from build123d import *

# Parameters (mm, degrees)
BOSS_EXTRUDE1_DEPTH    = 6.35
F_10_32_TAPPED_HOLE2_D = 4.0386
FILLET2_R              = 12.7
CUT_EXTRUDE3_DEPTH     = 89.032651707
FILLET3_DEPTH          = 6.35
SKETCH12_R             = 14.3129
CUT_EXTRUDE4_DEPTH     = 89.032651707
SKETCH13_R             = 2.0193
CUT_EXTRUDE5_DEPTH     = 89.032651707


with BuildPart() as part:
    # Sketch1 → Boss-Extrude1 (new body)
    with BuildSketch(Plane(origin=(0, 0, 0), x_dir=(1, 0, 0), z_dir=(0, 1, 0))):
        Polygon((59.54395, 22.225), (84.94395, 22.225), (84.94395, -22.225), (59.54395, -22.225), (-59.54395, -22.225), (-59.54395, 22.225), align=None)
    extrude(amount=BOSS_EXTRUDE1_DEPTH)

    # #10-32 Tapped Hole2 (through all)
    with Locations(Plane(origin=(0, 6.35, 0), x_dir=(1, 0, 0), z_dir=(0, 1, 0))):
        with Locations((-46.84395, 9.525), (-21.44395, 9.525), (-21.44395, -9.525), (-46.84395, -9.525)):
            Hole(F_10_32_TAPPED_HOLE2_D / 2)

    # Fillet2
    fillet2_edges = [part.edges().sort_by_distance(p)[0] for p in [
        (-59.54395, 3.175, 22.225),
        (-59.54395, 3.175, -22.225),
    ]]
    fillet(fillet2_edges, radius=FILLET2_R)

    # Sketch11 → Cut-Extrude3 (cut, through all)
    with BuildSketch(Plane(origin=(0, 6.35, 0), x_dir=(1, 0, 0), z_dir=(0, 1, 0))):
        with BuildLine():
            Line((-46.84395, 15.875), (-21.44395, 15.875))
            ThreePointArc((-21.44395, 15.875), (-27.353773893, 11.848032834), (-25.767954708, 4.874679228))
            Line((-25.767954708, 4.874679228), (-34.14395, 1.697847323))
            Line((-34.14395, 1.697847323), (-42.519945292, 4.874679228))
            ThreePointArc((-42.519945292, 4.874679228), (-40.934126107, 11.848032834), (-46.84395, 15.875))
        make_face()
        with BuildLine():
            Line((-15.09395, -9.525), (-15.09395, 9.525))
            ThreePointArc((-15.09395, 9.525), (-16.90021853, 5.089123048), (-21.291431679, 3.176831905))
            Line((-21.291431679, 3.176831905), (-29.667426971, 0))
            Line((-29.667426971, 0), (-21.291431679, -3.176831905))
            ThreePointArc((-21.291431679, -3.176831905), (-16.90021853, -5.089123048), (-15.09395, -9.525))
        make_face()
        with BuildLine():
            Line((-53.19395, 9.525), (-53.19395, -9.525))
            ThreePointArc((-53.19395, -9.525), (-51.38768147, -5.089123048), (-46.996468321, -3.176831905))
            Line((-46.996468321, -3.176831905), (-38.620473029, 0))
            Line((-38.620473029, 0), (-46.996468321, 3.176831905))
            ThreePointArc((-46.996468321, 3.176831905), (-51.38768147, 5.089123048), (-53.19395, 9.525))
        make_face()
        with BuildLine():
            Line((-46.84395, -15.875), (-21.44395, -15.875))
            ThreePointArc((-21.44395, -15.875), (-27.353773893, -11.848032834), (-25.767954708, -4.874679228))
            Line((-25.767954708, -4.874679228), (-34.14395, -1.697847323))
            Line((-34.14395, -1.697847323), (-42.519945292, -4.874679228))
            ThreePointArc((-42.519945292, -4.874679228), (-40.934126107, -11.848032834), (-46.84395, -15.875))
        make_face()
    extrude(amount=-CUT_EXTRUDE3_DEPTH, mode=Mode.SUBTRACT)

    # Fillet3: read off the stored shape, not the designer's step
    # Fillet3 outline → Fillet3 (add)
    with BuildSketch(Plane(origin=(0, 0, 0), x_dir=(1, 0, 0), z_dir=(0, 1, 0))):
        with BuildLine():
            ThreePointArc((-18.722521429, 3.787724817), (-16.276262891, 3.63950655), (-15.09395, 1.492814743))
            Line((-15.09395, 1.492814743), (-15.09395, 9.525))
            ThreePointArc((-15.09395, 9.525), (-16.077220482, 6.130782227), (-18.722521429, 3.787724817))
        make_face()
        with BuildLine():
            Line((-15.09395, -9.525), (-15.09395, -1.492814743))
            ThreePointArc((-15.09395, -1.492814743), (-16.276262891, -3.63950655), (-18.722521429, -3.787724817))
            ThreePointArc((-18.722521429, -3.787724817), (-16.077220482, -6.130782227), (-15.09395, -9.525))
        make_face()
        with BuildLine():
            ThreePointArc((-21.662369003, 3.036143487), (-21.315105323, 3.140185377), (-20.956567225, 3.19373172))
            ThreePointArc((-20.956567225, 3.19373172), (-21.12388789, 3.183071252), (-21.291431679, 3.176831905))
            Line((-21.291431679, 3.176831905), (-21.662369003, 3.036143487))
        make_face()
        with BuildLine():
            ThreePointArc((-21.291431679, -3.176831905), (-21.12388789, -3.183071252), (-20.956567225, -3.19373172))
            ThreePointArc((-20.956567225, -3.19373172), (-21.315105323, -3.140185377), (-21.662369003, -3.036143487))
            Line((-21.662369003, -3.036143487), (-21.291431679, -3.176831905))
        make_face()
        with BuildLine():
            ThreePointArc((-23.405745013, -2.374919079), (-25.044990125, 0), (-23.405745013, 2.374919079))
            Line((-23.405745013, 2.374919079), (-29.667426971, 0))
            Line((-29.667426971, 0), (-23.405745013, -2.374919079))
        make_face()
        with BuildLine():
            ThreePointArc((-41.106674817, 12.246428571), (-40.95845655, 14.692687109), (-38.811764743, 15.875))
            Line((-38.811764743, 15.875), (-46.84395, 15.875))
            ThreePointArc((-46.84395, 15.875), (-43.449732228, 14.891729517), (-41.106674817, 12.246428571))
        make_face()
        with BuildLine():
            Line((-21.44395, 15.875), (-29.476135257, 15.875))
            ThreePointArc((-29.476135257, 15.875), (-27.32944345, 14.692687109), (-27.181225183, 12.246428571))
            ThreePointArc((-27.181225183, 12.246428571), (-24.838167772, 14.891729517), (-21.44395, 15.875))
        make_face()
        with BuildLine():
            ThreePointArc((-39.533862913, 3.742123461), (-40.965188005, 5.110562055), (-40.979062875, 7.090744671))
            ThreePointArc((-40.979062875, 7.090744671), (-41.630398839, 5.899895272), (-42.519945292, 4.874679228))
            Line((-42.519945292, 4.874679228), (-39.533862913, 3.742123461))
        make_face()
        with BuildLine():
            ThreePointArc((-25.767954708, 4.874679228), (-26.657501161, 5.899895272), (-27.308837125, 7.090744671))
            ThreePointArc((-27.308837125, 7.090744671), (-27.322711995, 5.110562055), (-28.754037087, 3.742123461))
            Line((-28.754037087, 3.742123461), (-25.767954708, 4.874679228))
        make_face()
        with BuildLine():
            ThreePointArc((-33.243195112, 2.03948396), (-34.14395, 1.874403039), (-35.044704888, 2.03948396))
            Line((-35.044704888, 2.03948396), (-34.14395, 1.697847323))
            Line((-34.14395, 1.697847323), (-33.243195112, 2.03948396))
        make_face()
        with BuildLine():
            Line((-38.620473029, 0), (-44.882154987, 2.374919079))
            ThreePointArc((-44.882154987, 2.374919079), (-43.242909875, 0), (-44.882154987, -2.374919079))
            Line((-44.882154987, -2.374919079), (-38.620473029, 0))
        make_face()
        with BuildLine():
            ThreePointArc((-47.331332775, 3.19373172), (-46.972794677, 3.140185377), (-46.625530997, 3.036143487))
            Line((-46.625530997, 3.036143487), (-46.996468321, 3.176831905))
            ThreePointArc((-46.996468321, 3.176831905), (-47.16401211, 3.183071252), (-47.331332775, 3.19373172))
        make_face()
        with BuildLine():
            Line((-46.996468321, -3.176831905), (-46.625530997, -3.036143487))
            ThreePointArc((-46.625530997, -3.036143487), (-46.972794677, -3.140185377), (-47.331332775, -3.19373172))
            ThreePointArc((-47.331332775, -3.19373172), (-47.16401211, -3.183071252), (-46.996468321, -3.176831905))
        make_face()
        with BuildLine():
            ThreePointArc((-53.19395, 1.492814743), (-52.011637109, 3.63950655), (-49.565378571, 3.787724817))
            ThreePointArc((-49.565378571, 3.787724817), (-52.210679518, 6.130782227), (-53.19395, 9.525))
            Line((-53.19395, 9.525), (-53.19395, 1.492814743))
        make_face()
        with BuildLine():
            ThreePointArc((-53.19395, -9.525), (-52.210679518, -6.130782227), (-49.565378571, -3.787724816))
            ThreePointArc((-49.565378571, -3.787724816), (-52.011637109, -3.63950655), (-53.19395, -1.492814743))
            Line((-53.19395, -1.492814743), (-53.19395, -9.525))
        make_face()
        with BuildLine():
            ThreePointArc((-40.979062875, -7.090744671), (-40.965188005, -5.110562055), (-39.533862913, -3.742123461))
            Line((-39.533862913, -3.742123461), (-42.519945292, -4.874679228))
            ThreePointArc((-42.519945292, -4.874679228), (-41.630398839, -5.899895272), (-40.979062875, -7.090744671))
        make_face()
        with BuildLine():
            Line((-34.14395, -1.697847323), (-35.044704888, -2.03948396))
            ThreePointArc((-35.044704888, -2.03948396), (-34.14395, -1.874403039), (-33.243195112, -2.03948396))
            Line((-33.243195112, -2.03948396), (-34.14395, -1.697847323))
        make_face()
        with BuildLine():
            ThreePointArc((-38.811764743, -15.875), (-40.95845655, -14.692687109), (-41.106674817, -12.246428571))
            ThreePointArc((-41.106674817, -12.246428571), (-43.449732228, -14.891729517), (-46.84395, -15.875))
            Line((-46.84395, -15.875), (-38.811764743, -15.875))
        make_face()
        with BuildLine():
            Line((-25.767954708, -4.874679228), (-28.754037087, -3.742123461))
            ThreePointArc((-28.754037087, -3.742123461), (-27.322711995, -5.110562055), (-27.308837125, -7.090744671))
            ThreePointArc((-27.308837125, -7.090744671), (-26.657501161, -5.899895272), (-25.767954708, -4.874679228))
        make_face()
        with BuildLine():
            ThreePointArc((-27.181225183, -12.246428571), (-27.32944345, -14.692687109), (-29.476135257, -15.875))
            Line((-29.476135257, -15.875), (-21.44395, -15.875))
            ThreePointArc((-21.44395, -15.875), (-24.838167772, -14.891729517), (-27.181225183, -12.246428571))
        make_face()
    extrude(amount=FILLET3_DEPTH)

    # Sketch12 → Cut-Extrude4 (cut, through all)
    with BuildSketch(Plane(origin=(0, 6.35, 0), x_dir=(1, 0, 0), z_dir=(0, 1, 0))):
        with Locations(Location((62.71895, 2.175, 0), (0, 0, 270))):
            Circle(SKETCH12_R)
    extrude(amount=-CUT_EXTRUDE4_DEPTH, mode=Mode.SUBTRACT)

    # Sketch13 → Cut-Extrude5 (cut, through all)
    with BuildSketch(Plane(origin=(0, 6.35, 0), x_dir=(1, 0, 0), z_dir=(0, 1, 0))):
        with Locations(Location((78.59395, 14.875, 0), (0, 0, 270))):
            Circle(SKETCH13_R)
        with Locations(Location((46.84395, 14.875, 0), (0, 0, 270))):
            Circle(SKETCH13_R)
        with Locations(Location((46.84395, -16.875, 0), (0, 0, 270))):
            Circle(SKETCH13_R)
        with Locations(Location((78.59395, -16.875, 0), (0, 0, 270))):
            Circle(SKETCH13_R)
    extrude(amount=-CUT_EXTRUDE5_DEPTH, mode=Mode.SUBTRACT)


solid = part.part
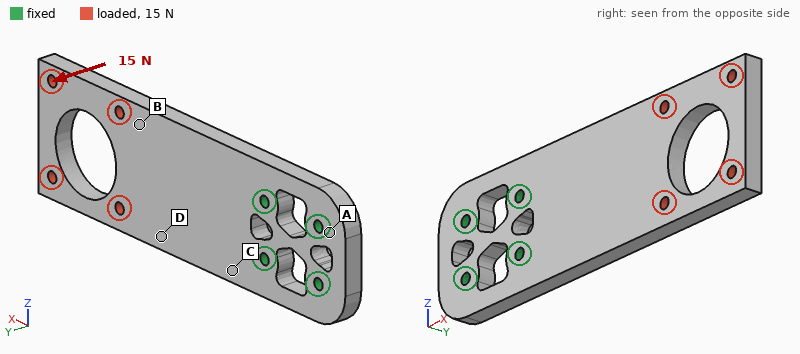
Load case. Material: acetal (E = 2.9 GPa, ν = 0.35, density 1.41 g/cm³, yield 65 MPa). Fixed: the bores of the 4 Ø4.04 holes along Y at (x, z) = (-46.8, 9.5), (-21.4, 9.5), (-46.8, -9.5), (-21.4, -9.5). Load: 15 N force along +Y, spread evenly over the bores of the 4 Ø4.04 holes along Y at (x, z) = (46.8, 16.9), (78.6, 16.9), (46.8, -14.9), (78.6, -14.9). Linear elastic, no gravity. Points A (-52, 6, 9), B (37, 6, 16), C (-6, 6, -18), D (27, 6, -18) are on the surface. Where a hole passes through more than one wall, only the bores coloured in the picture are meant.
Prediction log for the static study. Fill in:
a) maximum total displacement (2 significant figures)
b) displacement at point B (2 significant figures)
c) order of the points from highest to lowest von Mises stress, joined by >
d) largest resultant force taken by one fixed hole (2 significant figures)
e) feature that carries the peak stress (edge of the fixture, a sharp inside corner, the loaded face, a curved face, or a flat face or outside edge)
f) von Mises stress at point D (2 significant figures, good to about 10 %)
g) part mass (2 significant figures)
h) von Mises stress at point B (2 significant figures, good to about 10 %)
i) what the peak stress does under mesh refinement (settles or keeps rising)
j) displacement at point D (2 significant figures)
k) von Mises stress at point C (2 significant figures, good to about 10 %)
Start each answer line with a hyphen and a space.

- 1.7 mm
- 0.66 mm
- C > D > B > A
- 13 N
- edge of the fixture
- 1.8 MPa
- 46 g
- 1.4 MPa
- keeps rising
- 0.47 mm
- 3.5 MPa
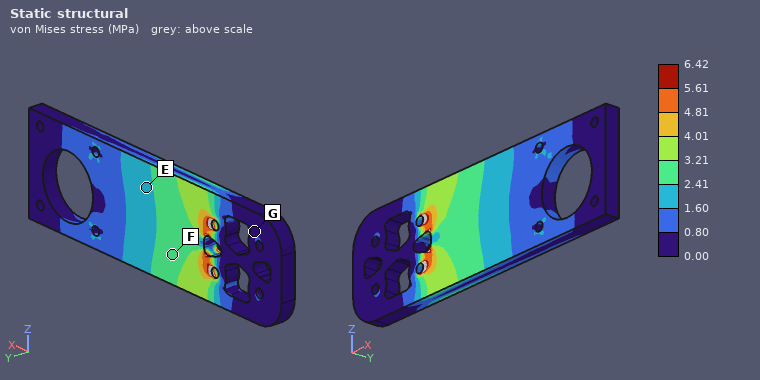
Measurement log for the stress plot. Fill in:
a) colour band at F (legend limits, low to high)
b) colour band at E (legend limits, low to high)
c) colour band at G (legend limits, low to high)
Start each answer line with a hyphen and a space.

- 2.41 to 3.21 MPa
- 1.60 to 2.41 MPa
- 0.00 to 0.80 MPa
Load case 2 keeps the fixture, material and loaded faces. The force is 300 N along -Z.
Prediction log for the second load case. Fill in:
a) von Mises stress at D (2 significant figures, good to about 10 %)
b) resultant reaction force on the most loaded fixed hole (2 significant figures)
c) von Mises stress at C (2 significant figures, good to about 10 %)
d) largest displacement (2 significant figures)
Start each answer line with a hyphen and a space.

- 4.1 MPa
- 810 N
- 7.3 MPa
- 1.2 mm
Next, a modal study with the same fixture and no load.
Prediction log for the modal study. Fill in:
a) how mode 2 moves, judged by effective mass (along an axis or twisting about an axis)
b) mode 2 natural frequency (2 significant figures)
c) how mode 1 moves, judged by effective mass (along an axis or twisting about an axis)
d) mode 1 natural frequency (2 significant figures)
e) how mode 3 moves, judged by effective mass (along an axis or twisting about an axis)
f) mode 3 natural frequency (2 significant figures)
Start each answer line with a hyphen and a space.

- twisting about X
- 600 Hz
- along Y
- 150 Hz
- along Y
- 720 Hz
